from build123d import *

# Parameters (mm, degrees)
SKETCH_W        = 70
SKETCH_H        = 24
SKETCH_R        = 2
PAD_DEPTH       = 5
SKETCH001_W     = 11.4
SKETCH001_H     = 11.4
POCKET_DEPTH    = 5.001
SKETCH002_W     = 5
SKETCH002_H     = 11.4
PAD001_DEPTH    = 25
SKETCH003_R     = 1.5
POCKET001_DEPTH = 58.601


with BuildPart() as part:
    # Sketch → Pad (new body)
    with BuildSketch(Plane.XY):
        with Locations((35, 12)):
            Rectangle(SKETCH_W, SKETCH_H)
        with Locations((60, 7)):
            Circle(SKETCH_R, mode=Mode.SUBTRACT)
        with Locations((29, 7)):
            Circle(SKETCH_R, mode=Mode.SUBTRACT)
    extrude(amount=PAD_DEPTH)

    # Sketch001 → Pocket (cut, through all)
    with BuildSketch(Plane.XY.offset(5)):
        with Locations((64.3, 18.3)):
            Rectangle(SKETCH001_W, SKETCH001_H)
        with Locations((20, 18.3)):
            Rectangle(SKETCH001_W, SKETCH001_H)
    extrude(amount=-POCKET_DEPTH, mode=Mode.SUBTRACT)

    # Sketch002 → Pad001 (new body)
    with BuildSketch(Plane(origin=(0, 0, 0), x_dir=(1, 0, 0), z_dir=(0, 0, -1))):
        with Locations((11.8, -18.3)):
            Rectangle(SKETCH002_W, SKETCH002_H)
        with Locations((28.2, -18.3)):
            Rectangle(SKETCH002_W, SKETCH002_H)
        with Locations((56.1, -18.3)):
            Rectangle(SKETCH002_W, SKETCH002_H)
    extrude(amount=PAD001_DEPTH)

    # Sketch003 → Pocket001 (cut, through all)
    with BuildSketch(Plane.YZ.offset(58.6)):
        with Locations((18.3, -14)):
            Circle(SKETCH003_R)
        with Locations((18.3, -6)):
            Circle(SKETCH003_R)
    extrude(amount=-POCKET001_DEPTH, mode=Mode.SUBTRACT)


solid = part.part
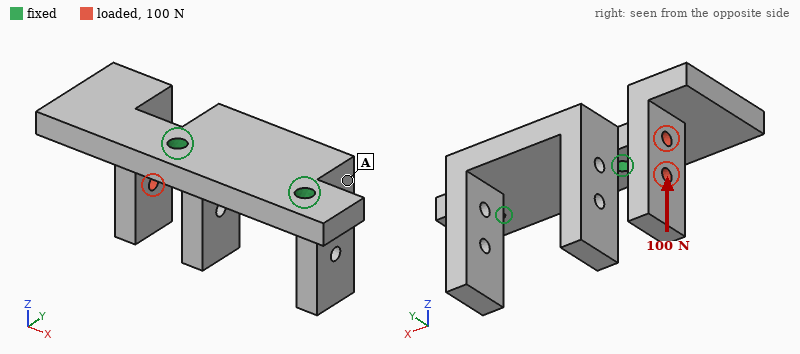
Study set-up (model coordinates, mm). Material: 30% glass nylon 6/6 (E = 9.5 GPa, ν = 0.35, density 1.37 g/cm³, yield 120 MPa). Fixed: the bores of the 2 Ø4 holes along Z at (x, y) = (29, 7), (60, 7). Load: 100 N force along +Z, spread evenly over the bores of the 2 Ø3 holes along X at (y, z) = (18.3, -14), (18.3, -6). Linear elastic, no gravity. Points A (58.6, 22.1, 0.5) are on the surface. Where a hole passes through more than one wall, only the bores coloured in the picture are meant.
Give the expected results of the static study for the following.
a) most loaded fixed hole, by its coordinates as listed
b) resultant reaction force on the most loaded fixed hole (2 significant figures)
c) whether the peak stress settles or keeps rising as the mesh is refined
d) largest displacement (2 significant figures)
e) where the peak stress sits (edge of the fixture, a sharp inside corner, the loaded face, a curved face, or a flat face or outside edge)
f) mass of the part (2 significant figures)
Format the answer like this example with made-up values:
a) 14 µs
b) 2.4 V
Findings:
a) (29, 7)
b) 110 N
c) keeps rising
d) 0.68 mm
e) edge of the fixture
f) 15 g
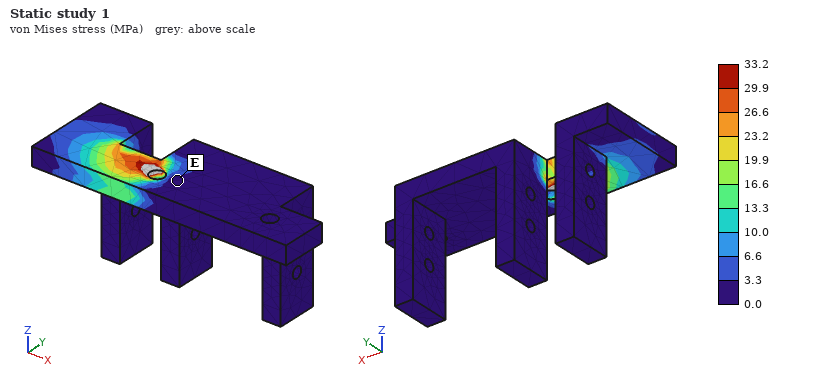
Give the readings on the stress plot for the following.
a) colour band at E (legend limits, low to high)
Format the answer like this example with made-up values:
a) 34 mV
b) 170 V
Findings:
a) 0.0 to 3.3 MPa
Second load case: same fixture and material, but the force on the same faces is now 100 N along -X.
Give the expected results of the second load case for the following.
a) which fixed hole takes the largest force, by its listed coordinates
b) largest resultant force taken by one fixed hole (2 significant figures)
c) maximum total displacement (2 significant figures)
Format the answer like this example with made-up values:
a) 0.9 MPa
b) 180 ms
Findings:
a) (29, 7)
b) 88 N
c) 0.85 mm
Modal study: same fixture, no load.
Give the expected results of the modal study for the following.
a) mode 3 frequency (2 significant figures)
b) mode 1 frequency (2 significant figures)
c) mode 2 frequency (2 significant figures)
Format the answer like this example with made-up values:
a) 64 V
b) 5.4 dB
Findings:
a) 2100 Hz
b) 1100 Hz
c) 1400 Hz
